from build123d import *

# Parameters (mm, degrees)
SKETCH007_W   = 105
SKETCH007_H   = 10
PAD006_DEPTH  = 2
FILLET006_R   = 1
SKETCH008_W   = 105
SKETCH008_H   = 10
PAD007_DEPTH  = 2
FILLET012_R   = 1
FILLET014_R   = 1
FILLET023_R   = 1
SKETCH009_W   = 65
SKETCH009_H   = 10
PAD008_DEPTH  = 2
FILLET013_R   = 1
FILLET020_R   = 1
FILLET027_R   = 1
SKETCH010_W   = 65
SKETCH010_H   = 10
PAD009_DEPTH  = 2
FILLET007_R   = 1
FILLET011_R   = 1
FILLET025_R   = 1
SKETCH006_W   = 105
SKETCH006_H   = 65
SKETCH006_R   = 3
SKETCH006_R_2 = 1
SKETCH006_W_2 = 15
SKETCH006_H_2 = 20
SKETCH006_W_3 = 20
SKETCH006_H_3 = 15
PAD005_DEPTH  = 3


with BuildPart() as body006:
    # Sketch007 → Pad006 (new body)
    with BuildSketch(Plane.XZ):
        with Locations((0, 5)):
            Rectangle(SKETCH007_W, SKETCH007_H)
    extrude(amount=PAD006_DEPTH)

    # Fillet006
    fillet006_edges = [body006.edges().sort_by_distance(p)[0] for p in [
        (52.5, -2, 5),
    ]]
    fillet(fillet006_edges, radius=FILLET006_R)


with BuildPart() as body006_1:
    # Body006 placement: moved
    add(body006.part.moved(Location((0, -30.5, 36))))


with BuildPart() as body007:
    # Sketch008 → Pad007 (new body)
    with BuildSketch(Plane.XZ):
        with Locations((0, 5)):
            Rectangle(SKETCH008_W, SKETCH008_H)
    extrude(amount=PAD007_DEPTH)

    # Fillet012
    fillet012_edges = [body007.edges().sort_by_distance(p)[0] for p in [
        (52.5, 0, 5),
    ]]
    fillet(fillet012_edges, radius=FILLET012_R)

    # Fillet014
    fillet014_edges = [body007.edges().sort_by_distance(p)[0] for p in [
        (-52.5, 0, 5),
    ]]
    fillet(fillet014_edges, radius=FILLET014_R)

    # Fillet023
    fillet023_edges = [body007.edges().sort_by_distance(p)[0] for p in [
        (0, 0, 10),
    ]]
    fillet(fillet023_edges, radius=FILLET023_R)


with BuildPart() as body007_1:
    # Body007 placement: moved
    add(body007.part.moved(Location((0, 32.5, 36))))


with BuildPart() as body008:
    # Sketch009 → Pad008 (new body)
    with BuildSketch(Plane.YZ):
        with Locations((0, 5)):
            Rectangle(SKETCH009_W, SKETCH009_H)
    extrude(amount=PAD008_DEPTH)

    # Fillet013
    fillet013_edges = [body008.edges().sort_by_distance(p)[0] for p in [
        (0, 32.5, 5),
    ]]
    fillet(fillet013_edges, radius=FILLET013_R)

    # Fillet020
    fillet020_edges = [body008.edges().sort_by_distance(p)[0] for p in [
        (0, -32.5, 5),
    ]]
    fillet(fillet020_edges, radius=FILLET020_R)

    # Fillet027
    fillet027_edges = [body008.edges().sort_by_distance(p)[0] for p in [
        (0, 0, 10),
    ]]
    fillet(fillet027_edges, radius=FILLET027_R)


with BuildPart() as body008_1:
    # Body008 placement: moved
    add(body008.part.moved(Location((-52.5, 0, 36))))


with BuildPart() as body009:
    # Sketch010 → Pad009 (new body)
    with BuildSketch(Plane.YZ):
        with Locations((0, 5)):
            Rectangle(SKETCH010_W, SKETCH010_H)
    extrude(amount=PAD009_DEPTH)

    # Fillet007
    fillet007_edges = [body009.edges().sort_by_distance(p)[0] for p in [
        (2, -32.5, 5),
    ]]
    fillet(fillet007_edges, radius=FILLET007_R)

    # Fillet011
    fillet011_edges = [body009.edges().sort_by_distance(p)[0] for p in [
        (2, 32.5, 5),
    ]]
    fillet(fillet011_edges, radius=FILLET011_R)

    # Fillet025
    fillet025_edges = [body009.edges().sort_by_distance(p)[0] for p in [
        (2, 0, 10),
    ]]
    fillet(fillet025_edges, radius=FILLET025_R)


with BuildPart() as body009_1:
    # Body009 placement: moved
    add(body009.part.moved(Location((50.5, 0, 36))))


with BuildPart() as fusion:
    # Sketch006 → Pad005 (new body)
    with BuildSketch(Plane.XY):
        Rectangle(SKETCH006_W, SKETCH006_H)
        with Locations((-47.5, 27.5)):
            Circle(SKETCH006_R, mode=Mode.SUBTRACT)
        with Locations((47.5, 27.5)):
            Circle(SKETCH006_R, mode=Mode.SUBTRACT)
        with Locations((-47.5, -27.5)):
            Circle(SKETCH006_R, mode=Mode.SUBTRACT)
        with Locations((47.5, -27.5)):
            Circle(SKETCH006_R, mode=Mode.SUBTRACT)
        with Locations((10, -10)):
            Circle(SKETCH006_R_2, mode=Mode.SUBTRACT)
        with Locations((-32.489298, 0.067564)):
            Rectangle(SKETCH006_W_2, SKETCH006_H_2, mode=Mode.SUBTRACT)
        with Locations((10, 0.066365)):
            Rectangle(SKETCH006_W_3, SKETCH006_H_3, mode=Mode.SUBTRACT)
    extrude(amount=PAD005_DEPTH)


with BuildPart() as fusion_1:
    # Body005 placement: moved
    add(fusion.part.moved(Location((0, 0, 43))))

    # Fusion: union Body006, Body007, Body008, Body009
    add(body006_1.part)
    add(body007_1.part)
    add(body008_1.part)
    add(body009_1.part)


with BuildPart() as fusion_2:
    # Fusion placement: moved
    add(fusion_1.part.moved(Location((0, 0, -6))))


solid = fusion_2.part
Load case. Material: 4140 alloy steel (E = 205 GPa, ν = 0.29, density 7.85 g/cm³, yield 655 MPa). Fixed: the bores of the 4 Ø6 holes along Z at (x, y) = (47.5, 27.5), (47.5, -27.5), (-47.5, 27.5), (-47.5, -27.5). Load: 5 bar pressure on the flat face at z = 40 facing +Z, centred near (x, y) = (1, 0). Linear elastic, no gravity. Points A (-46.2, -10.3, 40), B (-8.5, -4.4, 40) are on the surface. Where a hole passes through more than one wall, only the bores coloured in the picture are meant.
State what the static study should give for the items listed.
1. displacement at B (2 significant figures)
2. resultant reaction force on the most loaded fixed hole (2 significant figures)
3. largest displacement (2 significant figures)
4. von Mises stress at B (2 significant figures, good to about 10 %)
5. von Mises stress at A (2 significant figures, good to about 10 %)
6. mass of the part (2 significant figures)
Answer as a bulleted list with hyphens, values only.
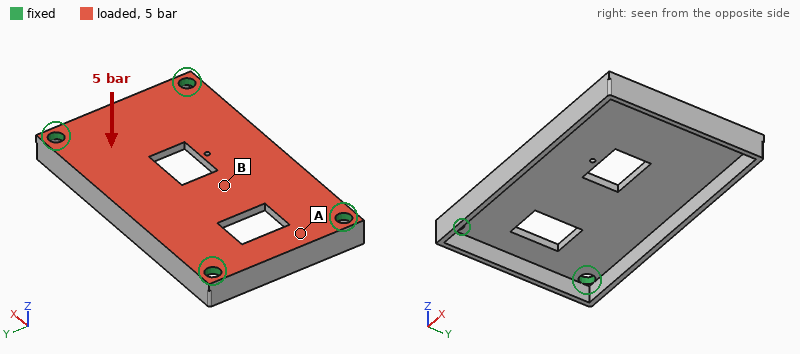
- 0.14 mm
- 800 N
- 0.16 mm
- 84 MPa
- 46 MPa
- 180 g
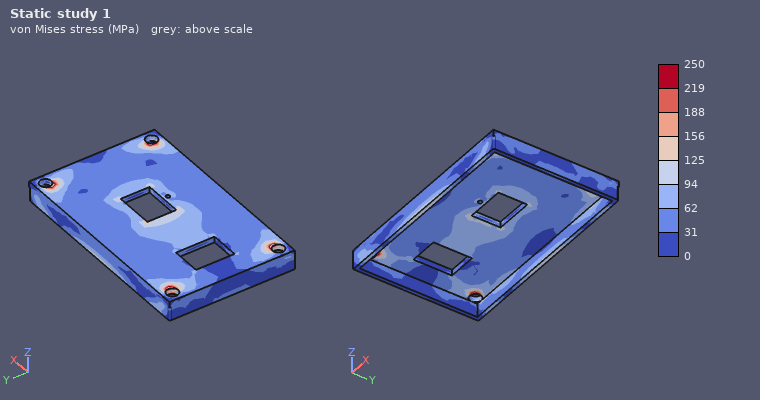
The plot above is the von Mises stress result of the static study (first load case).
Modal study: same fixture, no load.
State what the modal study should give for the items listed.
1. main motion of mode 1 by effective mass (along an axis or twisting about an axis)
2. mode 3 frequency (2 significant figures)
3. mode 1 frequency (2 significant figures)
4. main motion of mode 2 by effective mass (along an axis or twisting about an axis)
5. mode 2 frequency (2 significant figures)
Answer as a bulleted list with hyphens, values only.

- along Z
- 4900 Hz
- 2400 Hz
- twisting about X
- 4000 Hz
